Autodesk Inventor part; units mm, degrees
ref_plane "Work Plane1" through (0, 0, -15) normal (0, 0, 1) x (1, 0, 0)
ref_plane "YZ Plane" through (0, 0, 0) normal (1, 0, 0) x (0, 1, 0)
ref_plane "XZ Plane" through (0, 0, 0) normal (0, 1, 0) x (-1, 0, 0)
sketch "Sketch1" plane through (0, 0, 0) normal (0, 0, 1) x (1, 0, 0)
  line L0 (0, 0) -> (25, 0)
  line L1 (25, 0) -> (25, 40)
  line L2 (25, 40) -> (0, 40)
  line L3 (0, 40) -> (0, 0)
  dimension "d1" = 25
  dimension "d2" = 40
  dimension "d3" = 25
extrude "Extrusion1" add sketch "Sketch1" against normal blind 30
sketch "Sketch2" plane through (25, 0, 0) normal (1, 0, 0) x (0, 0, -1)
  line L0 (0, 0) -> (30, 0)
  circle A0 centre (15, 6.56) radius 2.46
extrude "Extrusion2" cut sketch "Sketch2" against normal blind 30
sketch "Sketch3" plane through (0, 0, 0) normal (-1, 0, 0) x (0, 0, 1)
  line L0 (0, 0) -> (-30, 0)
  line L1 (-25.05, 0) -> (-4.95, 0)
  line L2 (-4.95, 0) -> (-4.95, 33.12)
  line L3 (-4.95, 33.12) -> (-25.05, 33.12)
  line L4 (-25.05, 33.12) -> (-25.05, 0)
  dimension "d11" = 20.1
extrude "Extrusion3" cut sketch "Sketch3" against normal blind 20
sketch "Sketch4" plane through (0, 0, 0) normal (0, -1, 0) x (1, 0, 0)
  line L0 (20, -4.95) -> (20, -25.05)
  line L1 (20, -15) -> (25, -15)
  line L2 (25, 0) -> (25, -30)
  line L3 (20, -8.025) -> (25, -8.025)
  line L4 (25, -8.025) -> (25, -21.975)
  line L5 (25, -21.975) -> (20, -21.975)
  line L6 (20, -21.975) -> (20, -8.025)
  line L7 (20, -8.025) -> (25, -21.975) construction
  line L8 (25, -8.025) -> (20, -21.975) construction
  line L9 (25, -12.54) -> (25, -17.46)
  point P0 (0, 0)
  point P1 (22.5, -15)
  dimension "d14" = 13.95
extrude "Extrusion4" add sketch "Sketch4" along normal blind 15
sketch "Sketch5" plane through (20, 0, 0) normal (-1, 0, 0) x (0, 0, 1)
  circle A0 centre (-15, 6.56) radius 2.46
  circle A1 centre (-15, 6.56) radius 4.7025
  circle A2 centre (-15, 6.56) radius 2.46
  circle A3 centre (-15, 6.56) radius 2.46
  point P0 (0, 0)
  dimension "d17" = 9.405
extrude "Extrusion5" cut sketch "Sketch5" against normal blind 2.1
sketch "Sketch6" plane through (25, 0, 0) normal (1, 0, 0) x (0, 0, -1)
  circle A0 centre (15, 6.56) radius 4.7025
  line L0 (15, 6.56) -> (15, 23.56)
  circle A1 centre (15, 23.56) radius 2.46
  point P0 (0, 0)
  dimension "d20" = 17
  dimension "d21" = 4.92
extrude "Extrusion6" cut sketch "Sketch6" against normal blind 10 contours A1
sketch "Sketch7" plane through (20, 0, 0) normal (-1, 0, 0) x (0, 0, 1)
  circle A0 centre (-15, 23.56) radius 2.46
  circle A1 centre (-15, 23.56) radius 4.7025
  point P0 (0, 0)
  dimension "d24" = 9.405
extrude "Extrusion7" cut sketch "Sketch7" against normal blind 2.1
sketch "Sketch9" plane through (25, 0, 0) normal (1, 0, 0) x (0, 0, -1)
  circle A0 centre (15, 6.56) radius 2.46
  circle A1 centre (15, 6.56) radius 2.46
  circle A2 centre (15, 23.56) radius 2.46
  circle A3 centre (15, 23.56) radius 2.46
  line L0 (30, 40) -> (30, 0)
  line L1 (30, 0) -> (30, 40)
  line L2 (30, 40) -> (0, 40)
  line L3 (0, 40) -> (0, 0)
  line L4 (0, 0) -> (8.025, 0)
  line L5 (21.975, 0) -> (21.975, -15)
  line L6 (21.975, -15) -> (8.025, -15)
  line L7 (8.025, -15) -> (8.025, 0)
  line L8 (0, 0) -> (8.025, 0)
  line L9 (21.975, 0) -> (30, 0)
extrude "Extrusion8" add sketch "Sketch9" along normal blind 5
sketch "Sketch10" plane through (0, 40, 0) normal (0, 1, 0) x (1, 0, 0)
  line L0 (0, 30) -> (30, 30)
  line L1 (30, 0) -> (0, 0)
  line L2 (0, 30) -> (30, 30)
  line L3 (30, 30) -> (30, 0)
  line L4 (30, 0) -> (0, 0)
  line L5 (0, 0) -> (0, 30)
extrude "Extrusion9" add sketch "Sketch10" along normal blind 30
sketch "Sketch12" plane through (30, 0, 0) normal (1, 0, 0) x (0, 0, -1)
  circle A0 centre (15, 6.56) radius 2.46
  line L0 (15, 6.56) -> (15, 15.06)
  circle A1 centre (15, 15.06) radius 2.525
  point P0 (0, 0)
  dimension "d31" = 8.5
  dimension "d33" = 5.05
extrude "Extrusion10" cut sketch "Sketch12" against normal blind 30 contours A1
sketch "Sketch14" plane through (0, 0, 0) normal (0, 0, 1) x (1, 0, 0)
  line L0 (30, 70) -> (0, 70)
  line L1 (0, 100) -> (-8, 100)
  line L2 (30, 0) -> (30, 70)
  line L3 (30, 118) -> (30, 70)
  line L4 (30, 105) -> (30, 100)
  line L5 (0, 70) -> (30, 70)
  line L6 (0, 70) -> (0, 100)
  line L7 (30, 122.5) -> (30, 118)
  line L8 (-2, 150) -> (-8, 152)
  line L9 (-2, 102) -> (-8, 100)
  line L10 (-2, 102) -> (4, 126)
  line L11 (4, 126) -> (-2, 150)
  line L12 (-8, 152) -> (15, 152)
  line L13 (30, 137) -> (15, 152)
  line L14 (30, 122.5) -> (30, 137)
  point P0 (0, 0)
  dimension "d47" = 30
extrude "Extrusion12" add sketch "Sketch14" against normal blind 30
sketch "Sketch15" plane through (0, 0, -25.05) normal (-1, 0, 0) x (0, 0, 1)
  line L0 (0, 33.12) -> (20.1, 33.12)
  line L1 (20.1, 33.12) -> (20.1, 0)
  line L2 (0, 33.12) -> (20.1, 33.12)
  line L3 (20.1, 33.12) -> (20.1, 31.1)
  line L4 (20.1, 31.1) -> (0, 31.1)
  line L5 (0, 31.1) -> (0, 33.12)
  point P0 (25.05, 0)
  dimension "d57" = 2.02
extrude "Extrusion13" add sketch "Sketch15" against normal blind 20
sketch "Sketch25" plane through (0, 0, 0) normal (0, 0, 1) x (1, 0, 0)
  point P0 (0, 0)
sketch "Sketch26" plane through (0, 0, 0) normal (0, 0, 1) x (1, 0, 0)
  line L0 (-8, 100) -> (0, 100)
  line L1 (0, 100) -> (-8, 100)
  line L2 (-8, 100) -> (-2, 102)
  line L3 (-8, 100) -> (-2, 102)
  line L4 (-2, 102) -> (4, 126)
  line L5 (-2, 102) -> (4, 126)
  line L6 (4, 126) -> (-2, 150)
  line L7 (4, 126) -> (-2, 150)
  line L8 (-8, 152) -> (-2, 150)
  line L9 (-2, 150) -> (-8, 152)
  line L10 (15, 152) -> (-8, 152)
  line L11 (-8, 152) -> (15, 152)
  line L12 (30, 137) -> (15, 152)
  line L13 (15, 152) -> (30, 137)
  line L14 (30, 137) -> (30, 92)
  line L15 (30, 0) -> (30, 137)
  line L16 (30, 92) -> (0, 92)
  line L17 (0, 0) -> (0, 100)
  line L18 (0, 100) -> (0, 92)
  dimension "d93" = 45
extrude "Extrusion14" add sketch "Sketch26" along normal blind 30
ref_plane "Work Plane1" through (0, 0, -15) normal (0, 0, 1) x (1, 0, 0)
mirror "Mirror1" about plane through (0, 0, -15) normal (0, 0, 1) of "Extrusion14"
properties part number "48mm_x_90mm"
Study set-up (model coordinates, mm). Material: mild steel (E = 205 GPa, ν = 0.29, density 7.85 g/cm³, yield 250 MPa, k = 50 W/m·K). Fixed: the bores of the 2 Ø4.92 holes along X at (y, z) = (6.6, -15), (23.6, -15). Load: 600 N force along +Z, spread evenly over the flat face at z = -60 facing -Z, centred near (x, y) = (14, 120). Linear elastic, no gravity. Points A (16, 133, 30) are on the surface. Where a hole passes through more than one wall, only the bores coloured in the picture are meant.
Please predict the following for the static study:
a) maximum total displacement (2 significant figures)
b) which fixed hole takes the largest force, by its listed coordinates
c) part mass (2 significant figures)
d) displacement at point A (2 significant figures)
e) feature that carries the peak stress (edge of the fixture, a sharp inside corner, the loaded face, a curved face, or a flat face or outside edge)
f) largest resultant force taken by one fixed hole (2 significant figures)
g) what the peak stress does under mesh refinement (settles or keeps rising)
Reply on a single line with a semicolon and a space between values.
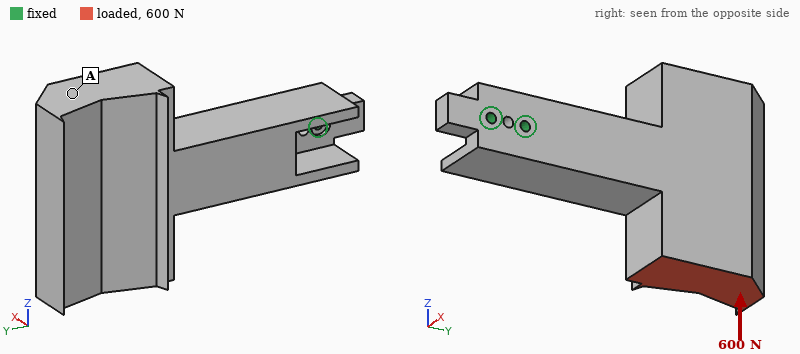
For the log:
58 µm; (23.6, -15); 1.7 kg; 50 µm; edge of the fixture; 3.1 kN; keeps rising
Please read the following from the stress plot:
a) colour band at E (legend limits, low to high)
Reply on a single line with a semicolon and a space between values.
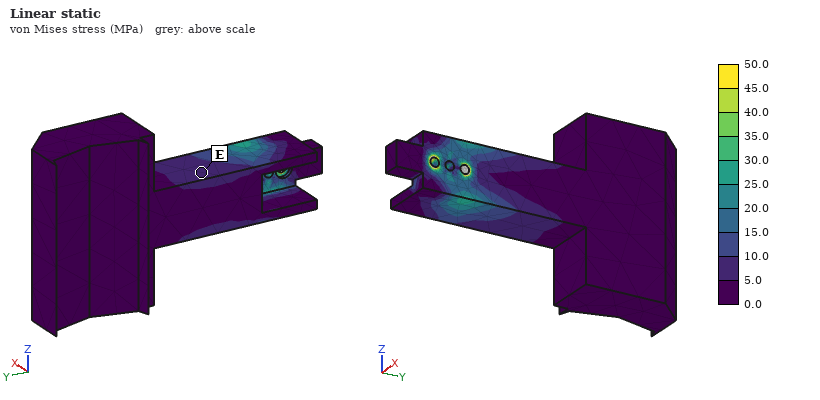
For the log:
5.0 to 10.0 MPa
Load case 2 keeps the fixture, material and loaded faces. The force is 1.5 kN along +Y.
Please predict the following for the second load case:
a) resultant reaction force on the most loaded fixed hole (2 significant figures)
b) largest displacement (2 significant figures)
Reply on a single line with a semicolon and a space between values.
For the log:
3.1 kN; 85 µm
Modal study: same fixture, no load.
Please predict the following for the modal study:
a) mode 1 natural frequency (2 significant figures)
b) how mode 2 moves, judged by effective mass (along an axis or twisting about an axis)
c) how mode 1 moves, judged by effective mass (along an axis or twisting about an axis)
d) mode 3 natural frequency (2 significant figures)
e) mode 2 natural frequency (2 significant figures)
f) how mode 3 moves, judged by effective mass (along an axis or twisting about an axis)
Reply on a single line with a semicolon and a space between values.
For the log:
470 Hz; along Z; along X; 1100 Hz; 530 Hz; twisting about Y
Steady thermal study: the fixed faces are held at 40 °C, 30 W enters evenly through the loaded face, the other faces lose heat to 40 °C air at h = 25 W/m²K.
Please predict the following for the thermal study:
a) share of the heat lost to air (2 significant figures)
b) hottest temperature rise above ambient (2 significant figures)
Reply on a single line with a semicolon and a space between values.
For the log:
62 %; 44 K
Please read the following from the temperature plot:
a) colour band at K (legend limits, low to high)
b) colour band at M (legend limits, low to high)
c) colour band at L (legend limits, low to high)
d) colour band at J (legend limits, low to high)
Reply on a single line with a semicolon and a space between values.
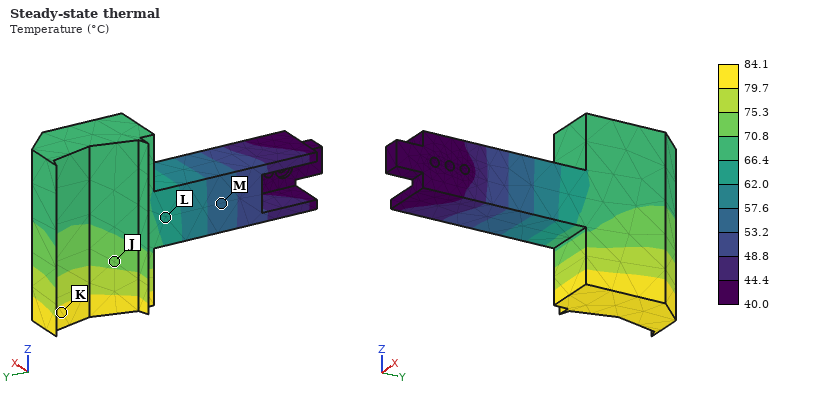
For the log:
79.7 to 84.1 °C; 53.2 to 57.6 °C; 62.0 to 66.4 °C; 70.8 to 75.3 °C
